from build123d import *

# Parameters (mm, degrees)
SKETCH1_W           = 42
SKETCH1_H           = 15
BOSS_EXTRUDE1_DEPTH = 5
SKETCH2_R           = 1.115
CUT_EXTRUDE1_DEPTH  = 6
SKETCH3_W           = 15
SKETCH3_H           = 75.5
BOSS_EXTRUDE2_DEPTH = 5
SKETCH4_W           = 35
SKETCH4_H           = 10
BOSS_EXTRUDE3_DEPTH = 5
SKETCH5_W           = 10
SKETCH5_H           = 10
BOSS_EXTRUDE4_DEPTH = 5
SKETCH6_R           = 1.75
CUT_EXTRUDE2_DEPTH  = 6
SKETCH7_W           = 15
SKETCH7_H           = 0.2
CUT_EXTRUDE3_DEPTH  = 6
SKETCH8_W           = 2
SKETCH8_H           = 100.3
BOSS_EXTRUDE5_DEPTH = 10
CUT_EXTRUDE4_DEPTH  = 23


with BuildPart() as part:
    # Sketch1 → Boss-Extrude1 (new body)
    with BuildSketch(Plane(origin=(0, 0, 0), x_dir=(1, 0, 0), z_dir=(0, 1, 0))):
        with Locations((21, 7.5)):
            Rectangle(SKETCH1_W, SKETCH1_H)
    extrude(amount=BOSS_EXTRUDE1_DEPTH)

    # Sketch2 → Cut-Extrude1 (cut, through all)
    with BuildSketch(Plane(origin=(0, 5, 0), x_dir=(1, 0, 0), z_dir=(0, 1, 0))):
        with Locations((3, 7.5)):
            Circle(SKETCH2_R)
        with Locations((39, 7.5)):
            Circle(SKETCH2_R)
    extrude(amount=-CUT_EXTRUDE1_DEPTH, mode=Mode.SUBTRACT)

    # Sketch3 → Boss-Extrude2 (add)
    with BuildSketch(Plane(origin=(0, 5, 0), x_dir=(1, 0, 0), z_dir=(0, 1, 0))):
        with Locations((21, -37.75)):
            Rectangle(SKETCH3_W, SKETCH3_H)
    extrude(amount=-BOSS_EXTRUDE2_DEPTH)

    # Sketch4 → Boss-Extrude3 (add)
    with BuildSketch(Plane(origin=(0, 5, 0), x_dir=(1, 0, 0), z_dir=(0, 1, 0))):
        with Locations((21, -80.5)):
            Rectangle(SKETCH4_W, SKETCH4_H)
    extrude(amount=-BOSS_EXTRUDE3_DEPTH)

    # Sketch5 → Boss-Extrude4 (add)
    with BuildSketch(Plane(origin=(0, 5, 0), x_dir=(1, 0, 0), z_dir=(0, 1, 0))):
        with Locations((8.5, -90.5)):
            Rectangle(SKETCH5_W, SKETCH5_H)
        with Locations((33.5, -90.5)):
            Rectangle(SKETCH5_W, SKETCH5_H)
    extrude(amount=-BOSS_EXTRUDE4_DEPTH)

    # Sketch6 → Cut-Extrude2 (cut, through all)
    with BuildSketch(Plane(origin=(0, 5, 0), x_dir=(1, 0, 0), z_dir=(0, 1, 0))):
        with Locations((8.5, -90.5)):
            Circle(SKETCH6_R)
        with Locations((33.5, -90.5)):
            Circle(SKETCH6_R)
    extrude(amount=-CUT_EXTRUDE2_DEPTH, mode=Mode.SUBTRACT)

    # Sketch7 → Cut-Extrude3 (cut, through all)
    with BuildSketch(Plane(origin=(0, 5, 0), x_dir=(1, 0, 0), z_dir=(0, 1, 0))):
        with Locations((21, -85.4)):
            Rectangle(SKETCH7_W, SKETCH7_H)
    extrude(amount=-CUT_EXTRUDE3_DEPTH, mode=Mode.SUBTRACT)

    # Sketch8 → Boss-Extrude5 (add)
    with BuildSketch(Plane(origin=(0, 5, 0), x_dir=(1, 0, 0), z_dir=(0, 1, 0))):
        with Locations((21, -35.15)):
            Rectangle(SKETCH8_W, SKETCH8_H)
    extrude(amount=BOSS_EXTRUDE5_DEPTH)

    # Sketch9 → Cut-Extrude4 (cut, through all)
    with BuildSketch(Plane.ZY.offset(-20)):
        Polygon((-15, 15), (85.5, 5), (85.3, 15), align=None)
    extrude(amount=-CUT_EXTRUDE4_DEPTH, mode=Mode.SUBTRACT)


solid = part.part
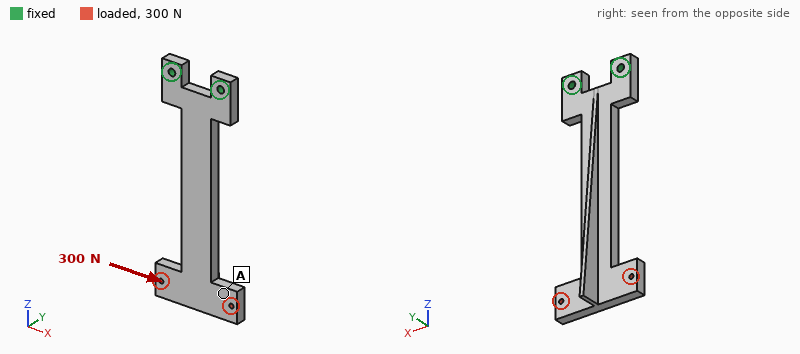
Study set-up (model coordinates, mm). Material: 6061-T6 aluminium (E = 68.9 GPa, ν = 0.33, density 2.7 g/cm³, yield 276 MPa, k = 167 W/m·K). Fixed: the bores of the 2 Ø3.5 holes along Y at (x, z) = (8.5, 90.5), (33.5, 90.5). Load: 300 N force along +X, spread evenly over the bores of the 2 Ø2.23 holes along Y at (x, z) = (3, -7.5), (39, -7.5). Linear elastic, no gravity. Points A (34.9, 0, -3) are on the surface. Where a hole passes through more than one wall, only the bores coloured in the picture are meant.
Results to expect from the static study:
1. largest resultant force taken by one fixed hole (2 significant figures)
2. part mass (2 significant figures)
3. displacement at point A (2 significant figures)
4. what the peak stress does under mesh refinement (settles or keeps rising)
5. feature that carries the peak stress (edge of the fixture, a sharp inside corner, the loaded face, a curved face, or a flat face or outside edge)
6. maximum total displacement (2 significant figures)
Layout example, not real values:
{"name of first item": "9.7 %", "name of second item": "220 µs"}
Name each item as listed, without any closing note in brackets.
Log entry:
{"largest resultant force taken by one fixed hole": "1.2 kN", "part mass": "34 g", "displacement at point A": "0.71 mm", "what the peak stress does under mesh refinement": "keeps rising", "feature that carries the peak stress": "a sharp inside corner", "maximum total displacement": "0.87 mm"}
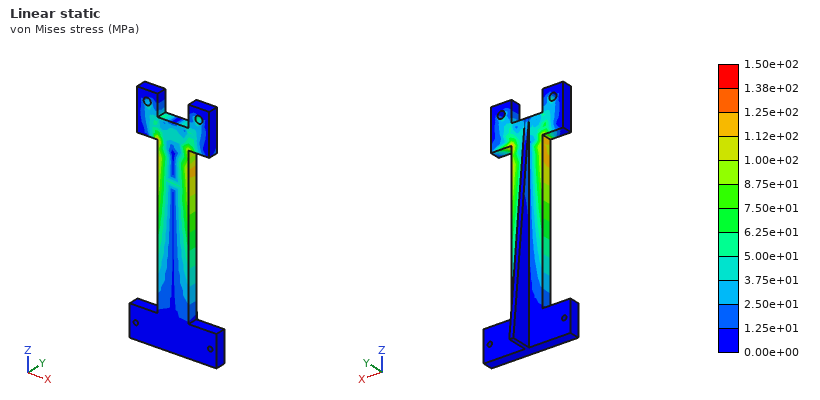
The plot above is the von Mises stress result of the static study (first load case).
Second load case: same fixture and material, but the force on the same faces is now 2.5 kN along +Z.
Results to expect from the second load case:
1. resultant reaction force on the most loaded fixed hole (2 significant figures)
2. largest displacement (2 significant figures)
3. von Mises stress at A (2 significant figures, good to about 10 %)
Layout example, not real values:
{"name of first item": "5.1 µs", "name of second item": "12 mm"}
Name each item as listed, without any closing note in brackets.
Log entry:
{"resultant reaction force on the most loaded fixed hole": "1.4 kN", "largest displacement": "0.18 mm", "von Mises stress at A": "34 MPa"}
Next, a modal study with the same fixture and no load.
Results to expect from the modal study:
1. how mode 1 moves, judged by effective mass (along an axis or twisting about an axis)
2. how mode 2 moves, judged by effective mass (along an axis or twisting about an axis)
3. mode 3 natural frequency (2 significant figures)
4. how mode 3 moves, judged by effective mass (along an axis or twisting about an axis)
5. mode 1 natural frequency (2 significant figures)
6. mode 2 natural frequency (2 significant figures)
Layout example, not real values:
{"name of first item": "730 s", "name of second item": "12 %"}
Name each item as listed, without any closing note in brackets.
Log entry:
{"how mode 1 moves, judged by effective mass": "along Y", "how mode 2 moves, judged by effective mass": "along X", "mode 3 natural frequency": "1700 Hz", "how mode 3 moves, judged by effective mass": "twisting about Z", "mode 1 natural frequency": "300 Hz", "mode 2 natural frequency": "890 Hz"}
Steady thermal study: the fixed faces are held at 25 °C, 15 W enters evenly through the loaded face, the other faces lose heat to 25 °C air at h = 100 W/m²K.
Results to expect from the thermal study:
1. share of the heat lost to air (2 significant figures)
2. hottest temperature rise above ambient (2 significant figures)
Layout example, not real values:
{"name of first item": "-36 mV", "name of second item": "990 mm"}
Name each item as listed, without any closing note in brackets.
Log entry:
{"share of the heat lost to air": "81 %", "hottest temperature rise above ambient": "39 K"}
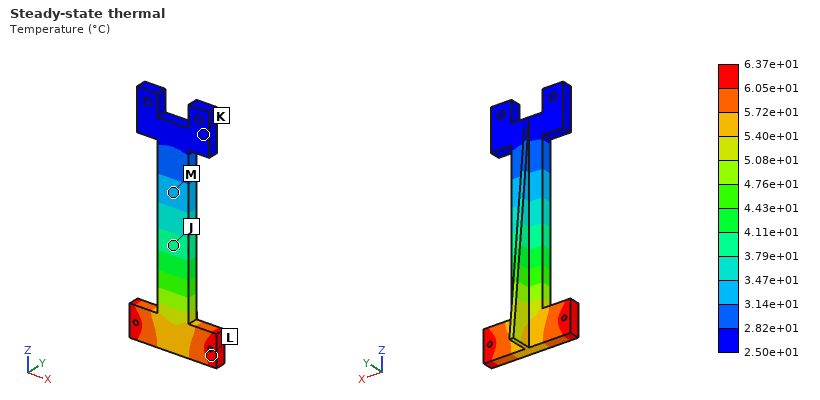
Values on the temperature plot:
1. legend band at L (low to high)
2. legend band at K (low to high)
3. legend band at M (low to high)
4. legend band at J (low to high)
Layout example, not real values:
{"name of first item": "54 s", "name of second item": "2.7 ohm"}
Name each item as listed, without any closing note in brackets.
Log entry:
{"legend band at L": "6.05e+01 to 6.37e+01 °C", "legend band at K": "2.50e+01 to 2.82e+01 °C", "legend band at M": "3.14e+01 to 3.47e+01 °C", "legend band at J": "3.79e+01 to 4.11e+01 °C"}
